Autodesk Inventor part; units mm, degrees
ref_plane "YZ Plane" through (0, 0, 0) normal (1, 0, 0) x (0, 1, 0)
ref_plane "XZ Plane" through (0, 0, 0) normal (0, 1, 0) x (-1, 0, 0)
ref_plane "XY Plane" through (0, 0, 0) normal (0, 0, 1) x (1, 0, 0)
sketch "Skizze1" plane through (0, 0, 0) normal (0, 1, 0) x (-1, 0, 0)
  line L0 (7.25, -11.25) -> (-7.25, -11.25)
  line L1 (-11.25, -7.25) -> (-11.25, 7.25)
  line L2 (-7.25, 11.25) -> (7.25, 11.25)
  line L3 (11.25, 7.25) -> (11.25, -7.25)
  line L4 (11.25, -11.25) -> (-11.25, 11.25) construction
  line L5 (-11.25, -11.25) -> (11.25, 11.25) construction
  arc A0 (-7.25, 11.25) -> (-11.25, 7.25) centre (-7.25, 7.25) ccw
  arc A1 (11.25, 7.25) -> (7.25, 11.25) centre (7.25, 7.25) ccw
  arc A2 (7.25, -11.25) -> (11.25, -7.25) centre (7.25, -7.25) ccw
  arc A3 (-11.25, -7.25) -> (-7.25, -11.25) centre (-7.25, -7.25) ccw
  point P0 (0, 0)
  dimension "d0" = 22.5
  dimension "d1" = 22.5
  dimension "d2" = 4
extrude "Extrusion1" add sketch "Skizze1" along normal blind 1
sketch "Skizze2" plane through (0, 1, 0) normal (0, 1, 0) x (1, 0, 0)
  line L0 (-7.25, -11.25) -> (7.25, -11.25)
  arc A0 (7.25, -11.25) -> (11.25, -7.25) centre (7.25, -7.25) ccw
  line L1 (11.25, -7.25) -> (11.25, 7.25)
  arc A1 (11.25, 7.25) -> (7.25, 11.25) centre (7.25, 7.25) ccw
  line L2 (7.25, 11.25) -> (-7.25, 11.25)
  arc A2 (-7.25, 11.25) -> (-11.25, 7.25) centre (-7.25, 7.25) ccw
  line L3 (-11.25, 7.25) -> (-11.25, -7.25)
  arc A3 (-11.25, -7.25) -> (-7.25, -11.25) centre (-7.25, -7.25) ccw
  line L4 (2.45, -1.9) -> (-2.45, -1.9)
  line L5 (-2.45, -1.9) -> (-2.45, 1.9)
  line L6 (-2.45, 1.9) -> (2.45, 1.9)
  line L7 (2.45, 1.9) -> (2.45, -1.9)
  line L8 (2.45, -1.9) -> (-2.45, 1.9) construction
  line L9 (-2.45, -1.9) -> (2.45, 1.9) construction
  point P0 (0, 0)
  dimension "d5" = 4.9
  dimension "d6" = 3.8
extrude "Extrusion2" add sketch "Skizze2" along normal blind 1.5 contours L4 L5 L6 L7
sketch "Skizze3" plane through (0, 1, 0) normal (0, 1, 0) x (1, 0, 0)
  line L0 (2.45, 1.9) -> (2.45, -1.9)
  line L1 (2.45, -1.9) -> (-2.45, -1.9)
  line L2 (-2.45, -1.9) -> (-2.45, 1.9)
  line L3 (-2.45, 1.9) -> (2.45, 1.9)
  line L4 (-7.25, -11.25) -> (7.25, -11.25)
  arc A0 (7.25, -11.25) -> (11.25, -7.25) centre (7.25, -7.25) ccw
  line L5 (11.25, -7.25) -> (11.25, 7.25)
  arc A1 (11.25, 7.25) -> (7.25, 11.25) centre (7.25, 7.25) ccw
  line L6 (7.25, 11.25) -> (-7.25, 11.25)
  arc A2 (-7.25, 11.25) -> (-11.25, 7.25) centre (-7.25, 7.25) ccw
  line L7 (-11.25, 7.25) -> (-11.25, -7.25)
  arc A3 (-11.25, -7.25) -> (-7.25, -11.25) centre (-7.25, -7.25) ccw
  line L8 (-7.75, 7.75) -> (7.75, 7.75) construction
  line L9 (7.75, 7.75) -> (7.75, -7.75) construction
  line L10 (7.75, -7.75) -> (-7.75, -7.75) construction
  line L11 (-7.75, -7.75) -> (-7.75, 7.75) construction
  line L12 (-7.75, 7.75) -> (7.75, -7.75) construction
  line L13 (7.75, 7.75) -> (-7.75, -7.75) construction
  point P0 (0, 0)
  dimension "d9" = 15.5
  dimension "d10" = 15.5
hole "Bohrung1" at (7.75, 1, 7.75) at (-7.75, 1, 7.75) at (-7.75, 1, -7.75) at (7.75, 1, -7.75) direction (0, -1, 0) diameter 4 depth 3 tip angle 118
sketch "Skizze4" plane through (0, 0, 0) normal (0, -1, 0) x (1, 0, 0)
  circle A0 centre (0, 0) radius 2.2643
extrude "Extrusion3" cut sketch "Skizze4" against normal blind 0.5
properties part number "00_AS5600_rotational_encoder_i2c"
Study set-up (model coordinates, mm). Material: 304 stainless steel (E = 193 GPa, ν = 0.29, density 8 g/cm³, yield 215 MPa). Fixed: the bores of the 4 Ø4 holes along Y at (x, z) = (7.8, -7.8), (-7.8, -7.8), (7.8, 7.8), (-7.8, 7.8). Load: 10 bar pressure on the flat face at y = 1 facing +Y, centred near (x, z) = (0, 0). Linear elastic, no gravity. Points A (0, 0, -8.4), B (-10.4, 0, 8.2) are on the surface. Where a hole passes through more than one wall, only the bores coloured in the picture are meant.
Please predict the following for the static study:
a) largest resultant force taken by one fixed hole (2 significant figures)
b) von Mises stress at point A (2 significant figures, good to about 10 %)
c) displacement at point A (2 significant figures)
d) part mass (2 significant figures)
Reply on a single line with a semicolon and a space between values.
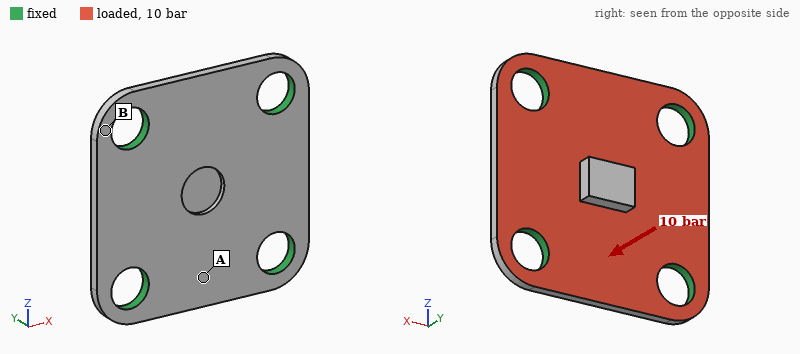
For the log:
110 N; 41 MPa; 4.2 µm; 3.7 g
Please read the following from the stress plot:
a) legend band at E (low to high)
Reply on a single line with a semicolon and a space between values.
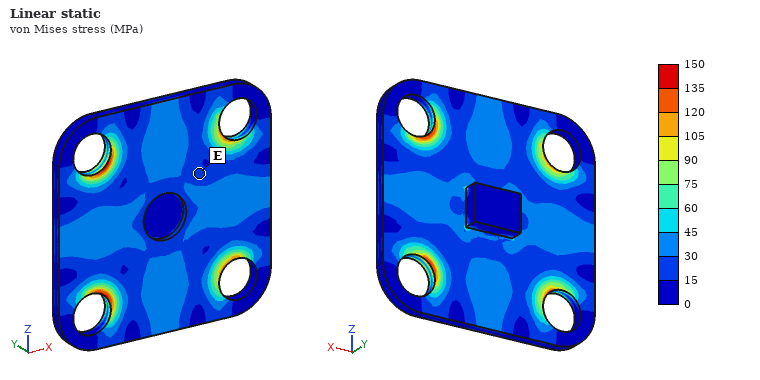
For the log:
15 to 30 MPa
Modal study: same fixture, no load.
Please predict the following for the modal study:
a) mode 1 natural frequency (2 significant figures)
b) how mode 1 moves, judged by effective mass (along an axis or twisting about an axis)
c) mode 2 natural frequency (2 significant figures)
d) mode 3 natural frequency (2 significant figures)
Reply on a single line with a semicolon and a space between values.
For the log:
20 kHz; along Y; 33 kHz; 33 kHz
